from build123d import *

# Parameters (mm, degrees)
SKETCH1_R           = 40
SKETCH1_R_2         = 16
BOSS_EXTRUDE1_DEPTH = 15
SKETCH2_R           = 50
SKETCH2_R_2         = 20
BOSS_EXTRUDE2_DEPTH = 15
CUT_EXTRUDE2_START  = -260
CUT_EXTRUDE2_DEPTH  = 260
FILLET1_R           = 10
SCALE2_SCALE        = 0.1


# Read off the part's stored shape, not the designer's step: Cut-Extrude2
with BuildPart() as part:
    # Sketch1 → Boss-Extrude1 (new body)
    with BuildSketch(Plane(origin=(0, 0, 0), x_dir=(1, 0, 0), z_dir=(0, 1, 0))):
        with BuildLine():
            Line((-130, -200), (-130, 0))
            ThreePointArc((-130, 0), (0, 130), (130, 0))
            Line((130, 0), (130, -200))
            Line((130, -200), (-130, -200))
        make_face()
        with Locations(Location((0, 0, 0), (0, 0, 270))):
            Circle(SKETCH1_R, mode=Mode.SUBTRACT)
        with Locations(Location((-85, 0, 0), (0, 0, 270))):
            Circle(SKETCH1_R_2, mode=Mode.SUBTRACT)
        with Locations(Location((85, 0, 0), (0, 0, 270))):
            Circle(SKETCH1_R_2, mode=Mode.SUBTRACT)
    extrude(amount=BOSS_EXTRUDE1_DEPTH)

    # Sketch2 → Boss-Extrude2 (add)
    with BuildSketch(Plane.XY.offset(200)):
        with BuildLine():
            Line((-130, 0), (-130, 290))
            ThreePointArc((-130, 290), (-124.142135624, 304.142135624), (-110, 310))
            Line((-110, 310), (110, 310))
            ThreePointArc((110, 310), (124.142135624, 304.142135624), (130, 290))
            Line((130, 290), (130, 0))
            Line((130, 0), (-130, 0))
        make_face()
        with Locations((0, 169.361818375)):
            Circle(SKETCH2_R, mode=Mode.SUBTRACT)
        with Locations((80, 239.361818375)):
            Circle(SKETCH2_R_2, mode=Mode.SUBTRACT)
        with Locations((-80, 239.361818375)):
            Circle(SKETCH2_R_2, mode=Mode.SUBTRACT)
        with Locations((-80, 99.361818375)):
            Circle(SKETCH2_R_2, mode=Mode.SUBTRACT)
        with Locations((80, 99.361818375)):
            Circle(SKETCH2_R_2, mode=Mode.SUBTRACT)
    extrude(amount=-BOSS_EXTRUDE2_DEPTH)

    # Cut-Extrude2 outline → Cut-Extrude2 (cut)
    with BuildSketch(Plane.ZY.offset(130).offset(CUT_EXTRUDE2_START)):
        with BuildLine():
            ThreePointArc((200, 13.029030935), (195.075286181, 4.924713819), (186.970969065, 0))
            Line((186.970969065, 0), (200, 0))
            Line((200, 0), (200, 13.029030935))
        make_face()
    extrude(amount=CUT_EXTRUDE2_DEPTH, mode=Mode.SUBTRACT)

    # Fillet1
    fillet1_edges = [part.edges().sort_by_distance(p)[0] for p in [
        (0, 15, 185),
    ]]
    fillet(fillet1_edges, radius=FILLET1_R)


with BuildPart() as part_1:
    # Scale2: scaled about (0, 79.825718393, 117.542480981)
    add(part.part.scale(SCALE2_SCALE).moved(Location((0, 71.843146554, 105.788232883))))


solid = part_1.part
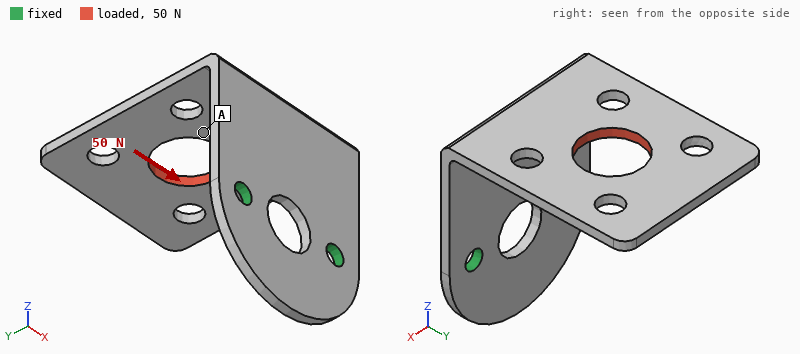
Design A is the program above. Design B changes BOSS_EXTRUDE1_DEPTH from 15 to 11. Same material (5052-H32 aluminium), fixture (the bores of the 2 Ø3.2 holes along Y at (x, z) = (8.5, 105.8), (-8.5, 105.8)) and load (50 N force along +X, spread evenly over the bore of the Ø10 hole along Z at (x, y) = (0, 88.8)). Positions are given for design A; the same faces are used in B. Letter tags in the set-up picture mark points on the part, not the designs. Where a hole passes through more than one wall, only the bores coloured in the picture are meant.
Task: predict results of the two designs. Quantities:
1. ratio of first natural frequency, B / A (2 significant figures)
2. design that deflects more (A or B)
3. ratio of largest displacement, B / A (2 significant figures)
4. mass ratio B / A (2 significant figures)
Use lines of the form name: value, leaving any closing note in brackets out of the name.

ratio of first natural frequency, B / A: 0.67
design that deflects more: B
ratio of largest displacement, B / A: 2.2
mass ratio B / A: 0.87
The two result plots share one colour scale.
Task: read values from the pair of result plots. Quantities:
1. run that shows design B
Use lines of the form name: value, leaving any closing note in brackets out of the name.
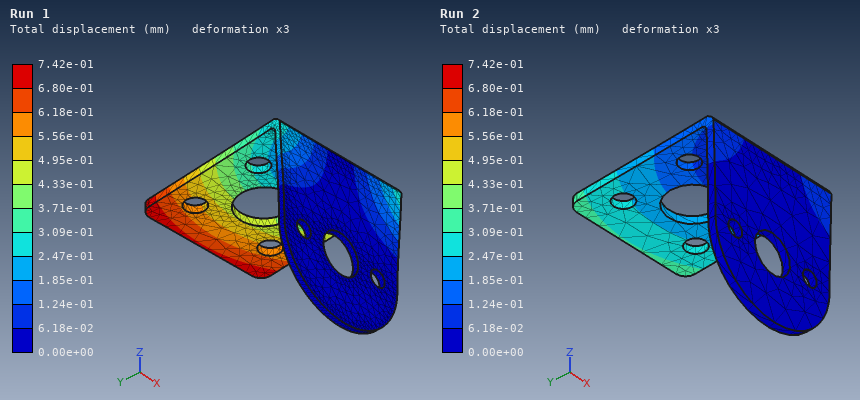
run that shows design B: Run 1
